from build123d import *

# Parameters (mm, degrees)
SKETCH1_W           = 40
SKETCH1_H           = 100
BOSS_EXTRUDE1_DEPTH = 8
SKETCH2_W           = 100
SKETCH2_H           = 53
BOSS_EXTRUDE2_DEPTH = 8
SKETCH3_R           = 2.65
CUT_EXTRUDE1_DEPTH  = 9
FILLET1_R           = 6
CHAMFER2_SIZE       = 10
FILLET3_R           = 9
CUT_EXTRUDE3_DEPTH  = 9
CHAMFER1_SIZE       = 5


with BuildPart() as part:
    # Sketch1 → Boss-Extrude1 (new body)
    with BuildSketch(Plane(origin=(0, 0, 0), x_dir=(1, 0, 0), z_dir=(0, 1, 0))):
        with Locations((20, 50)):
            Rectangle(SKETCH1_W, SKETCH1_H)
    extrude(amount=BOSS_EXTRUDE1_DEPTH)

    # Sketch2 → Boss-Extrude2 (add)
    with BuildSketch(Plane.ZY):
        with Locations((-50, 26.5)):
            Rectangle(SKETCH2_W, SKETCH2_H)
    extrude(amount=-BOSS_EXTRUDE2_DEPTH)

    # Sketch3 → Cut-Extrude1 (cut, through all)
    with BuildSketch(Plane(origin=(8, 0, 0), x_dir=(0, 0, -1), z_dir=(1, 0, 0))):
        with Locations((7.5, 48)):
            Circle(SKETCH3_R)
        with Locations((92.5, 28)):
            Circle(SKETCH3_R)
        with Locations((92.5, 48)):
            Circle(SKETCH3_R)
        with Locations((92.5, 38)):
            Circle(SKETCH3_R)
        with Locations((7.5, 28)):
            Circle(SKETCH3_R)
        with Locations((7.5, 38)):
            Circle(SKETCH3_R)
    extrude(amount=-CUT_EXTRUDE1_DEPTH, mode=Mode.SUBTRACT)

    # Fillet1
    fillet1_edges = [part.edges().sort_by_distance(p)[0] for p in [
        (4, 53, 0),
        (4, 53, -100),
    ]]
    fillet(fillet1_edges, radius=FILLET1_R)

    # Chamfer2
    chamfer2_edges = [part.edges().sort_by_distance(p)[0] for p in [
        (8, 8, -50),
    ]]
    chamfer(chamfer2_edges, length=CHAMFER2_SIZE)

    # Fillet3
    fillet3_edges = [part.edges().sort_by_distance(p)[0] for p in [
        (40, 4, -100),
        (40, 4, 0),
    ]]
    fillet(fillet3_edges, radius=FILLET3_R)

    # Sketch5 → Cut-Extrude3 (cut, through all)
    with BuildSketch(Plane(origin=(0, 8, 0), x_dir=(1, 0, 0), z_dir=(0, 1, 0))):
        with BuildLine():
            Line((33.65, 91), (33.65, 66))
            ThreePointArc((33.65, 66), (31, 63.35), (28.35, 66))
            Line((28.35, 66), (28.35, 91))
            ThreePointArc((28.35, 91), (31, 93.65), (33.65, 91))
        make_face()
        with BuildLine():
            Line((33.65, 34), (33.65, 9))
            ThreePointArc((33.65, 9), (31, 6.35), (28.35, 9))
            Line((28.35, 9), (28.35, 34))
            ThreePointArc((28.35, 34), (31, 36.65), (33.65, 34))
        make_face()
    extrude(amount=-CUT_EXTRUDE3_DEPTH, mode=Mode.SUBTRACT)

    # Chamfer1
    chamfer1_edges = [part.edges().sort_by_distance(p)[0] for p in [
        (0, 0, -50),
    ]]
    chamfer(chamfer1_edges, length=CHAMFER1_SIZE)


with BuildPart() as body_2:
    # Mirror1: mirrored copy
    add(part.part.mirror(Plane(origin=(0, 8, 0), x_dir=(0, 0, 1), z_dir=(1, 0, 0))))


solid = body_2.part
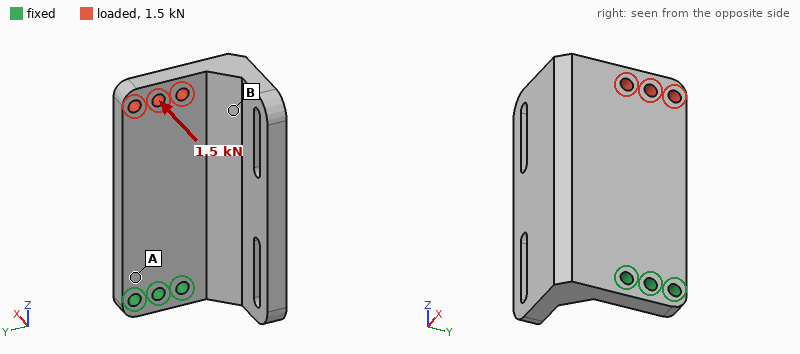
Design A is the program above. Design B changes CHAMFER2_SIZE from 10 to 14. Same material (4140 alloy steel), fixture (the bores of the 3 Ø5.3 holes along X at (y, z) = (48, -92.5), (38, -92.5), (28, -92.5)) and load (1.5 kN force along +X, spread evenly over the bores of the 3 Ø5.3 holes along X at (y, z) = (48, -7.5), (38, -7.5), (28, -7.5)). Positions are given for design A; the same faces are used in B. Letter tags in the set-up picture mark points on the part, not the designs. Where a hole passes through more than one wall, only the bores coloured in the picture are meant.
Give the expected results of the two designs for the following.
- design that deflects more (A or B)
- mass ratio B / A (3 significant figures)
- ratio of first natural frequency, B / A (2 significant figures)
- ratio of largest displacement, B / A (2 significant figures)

A
1.07
1.0
0.87
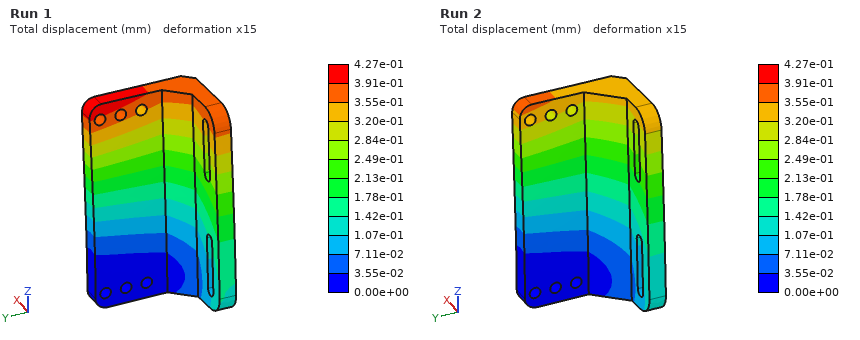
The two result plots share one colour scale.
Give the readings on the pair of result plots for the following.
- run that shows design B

Run 2
